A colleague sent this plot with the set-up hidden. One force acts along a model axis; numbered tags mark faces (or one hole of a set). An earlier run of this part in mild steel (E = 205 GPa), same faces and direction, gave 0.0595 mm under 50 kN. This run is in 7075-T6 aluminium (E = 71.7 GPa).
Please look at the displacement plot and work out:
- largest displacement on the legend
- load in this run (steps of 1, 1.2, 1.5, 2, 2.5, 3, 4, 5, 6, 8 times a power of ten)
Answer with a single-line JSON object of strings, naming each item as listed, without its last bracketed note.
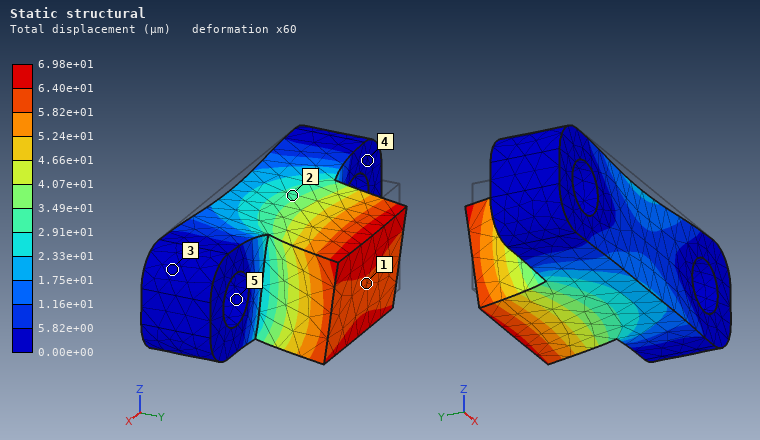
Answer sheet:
{"largest displacement on the legend": "6.98e+01 µm", "load in this run": "20 kN"}
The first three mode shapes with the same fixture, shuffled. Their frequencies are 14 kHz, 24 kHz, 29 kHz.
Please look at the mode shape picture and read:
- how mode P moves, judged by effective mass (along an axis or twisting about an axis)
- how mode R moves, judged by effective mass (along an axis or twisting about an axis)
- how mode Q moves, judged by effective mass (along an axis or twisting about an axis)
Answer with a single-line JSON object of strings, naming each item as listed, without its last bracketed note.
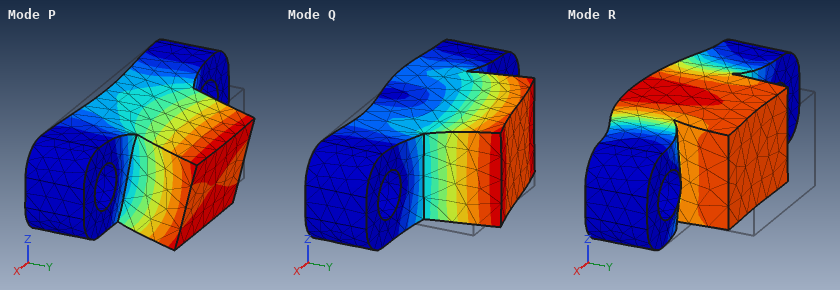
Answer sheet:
{"how mode P moves, judged by effective mass": "along Z", "how mode R moves, judged by effective mass": "along Y", "how mode Q moves, judged by effective mass": "along X"}
